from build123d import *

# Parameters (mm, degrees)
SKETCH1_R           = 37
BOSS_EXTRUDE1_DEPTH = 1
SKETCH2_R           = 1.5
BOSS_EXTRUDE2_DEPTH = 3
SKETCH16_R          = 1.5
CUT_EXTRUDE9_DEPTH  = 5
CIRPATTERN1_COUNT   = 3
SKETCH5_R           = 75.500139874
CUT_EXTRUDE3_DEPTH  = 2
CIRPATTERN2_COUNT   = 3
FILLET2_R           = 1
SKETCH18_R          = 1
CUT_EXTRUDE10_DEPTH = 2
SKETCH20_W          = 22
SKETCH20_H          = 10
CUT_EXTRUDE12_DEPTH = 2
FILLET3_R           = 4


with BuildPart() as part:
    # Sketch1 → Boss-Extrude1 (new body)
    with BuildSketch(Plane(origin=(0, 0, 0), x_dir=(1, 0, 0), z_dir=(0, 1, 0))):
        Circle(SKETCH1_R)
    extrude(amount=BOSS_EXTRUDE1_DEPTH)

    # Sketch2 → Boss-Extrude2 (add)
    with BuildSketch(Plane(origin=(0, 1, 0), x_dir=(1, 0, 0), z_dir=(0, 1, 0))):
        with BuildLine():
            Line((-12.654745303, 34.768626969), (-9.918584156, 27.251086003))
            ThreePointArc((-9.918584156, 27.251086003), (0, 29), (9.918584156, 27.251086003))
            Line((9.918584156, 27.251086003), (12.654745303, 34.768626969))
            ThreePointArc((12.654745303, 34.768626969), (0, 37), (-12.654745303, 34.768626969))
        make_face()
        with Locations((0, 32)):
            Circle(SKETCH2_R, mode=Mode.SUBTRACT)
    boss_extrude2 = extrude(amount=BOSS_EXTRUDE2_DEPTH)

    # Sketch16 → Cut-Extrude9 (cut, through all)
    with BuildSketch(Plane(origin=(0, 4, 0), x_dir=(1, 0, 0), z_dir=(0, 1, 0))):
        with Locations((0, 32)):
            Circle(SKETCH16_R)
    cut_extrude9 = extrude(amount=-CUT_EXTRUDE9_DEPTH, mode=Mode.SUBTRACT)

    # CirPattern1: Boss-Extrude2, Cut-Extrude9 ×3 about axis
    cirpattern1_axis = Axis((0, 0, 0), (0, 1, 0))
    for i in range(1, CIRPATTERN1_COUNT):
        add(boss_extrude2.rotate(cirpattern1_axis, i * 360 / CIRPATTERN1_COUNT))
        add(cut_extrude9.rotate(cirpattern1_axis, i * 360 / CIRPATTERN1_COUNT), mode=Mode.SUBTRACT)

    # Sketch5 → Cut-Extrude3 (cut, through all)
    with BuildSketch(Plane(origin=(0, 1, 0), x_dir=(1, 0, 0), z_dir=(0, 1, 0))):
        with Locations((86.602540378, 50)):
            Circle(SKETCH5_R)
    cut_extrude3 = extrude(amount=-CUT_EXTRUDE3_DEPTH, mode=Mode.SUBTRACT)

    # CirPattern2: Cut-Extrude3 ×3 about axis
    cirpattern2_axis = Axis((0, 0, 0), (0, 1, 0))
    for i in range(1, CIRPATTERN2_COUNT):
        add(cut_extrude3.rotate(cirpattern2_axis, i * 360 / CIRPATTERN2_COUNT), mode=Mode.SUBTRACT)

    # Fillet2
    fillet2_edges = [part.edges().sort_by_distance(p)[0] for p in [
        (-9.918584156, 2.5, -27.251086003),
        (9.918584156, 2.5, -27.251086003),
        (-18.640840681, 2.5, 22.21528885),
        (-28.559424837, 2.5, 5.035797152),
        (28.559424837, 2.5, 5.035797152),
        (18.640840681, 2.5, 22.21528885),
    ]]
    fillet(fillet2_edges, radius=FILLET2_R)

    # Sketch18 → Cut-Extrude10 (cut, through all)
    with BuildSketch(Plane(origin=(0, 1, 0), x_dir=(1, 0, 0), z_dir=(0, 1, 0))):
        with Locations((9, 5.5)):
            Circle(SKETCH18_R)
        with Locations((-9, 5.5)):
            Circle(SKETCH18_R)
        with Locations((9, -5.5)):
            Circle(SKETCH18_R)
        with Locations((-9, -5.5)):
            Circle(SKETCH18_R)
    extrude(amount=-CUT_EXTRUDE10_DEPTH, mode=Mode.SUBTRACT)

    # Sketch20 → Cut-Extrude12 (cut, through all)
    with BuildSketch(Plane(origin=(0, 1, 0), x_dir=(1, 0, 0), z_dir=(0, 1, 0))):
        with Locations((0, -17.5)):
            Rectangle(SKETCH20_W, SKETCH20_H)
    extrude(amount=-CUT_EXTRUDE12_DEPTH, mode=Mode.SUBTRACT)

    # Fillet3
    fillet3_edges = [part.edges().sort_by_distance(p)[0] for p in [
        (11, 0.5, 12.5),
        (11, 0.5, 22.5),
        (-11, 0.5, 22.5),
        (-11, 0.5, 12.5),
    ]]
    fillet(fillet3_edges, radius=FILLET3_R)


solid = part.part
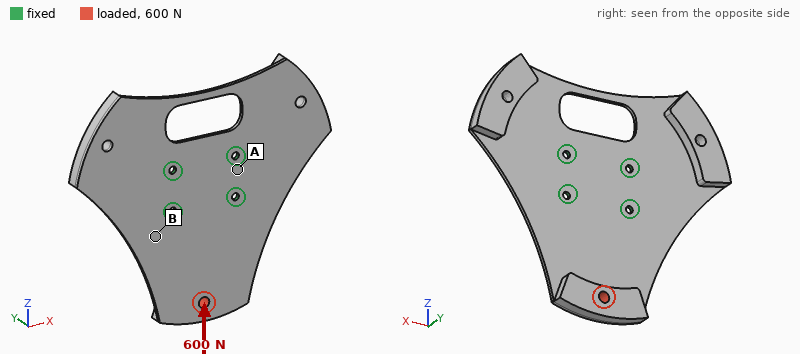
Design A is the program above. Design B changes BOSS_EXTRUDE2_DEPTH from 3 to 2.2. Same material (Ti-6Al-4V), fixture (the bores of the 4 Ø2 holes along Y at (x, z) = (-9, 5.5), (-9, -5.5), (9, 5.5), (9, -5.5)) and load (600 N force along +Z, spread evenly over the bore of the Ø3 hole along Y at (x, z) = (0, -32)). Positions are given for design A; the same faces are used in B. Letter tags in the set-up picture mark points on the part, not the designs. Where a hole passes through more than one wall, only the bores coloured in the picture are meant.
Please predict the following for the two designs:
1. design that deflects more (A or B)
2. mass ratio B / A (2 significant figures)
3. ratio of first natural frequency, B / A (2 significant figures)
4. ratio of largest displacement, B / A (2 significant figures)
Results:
A
0.90
1.1
0.73
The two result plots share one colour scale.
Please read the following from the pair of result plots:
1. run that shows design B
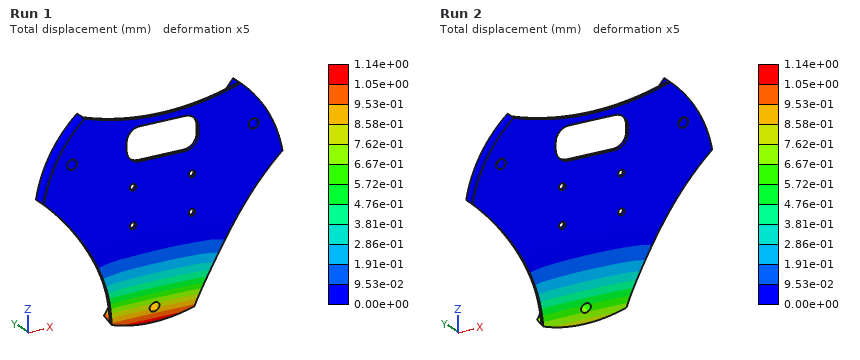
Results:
Run 2
